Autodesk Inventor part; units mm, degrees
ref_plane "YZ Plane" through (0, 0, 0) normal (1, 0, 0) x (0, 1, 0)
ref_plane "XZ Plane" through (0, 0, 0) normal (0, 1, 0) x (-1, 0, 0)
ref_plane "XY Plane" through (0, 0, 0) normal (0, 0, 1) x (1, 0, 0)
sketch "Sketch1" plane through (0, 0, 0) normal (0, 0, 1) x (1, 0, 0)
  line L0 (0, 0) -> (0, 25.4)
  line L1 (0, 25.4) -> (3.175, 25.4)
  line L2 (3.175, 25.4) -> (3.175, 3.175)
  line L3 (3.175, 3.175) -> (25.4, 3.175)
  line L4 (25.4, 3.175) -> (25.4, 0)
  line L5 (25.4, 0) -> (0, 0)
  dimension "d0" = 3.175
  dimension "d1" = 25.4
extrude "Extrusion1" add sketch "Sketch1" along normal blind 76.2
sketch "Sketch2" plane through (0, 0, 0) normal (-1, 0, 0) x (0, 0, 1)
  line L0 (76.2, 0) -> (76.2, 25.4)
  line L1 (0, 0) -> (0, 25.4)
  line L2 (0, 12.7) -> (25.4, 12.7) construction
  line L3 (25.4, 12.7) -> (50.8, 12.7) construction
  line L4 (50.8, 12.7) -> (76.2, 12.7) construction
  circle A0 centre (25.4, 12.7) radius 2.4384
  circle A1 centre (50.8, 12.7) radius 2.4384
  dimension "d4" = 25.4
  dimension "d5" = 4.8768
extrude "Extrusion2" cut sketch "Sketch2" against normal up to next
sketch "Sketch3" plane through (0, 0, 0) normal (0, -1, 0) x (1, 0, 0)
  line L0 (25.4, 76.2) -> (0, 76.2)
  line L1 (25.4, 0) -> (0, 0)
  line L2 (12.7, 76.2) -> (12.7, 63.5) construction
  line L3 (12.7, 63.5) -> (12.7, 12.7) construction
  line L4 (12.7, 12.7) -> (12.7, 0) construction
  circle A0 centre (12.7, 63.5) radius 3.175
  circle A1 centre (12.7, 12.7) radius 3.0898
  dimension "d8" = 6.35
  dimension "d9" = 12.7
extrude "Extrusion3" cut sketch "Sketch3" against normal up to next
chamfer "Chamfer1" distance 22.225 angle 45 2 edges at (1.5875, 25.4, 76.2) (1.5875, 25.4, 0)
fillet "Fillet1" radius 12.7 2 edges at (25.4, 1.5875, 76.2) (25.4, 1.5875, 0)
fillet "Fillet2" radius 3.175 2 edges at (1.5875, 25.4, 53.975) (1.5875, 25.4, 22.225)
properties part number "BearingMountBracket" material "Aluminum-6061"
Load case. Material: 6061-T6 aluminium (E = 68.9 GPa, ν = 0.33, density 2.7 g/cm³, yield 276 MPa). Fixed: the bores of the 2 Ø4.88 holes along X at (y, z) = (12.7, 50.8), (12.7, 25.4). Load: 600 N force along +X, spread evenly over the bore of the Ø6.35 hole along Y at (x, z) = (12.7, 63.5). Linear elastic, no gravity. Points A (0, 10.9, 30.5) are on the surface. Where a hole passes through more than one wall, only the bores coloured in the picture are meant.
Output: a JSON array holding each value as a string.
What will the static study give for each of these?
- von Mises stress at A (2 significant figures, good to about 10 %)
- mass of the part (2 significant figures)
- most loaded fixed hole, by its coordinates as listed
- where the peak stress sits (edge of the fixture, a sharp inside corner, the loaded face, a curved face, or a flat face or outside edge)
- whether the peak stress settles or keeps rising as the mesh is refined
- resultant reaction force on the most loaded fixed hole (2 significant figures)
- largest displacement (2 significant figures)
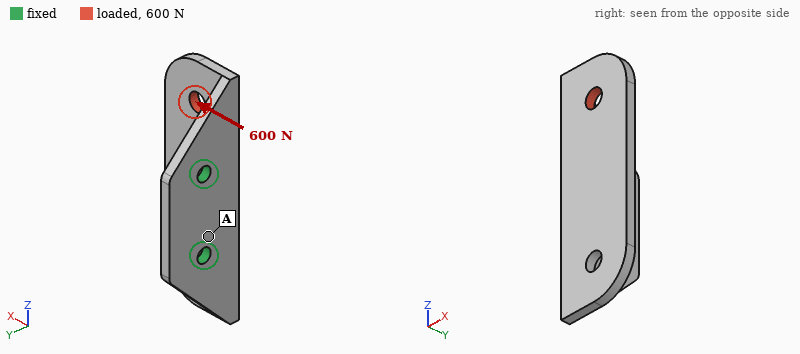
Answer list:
["23 MPa", "25 g", "(12.7, 50.8)", "edge of the fixture", "keeps rising", "800 N", "0.19 mm"]
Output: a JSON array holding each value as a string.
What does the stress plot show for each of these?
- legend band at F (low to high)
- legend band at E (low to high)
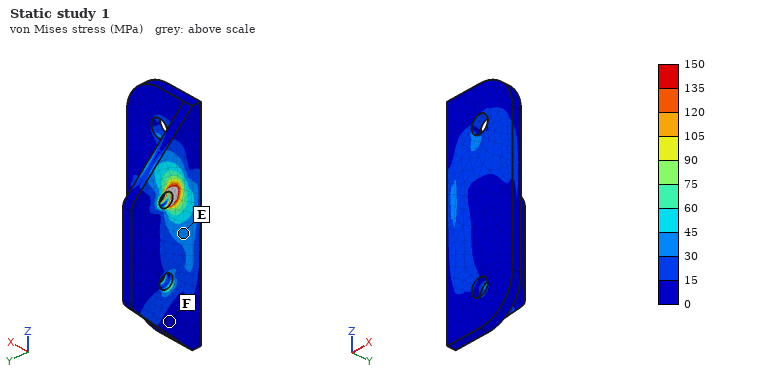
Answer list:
["0 to 15 MPa", "30 to 45 MPa"]
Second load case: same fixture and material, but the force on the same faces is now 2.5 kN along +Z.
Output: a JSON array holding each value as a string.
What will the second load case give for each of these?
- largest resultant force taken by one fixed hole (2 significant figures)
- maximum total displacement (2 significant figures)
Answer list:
["1.9 kN", "0.21 mm"]
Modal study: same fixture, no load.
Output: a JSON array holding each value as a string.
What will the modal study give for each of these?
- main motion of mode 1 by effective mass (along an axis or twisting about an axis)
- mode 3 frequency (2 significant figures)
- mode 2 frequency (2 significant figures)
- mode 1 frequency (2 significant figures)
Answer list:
["along Y", "5600 Hz", "3300 Hz", "2600 Hz"]
